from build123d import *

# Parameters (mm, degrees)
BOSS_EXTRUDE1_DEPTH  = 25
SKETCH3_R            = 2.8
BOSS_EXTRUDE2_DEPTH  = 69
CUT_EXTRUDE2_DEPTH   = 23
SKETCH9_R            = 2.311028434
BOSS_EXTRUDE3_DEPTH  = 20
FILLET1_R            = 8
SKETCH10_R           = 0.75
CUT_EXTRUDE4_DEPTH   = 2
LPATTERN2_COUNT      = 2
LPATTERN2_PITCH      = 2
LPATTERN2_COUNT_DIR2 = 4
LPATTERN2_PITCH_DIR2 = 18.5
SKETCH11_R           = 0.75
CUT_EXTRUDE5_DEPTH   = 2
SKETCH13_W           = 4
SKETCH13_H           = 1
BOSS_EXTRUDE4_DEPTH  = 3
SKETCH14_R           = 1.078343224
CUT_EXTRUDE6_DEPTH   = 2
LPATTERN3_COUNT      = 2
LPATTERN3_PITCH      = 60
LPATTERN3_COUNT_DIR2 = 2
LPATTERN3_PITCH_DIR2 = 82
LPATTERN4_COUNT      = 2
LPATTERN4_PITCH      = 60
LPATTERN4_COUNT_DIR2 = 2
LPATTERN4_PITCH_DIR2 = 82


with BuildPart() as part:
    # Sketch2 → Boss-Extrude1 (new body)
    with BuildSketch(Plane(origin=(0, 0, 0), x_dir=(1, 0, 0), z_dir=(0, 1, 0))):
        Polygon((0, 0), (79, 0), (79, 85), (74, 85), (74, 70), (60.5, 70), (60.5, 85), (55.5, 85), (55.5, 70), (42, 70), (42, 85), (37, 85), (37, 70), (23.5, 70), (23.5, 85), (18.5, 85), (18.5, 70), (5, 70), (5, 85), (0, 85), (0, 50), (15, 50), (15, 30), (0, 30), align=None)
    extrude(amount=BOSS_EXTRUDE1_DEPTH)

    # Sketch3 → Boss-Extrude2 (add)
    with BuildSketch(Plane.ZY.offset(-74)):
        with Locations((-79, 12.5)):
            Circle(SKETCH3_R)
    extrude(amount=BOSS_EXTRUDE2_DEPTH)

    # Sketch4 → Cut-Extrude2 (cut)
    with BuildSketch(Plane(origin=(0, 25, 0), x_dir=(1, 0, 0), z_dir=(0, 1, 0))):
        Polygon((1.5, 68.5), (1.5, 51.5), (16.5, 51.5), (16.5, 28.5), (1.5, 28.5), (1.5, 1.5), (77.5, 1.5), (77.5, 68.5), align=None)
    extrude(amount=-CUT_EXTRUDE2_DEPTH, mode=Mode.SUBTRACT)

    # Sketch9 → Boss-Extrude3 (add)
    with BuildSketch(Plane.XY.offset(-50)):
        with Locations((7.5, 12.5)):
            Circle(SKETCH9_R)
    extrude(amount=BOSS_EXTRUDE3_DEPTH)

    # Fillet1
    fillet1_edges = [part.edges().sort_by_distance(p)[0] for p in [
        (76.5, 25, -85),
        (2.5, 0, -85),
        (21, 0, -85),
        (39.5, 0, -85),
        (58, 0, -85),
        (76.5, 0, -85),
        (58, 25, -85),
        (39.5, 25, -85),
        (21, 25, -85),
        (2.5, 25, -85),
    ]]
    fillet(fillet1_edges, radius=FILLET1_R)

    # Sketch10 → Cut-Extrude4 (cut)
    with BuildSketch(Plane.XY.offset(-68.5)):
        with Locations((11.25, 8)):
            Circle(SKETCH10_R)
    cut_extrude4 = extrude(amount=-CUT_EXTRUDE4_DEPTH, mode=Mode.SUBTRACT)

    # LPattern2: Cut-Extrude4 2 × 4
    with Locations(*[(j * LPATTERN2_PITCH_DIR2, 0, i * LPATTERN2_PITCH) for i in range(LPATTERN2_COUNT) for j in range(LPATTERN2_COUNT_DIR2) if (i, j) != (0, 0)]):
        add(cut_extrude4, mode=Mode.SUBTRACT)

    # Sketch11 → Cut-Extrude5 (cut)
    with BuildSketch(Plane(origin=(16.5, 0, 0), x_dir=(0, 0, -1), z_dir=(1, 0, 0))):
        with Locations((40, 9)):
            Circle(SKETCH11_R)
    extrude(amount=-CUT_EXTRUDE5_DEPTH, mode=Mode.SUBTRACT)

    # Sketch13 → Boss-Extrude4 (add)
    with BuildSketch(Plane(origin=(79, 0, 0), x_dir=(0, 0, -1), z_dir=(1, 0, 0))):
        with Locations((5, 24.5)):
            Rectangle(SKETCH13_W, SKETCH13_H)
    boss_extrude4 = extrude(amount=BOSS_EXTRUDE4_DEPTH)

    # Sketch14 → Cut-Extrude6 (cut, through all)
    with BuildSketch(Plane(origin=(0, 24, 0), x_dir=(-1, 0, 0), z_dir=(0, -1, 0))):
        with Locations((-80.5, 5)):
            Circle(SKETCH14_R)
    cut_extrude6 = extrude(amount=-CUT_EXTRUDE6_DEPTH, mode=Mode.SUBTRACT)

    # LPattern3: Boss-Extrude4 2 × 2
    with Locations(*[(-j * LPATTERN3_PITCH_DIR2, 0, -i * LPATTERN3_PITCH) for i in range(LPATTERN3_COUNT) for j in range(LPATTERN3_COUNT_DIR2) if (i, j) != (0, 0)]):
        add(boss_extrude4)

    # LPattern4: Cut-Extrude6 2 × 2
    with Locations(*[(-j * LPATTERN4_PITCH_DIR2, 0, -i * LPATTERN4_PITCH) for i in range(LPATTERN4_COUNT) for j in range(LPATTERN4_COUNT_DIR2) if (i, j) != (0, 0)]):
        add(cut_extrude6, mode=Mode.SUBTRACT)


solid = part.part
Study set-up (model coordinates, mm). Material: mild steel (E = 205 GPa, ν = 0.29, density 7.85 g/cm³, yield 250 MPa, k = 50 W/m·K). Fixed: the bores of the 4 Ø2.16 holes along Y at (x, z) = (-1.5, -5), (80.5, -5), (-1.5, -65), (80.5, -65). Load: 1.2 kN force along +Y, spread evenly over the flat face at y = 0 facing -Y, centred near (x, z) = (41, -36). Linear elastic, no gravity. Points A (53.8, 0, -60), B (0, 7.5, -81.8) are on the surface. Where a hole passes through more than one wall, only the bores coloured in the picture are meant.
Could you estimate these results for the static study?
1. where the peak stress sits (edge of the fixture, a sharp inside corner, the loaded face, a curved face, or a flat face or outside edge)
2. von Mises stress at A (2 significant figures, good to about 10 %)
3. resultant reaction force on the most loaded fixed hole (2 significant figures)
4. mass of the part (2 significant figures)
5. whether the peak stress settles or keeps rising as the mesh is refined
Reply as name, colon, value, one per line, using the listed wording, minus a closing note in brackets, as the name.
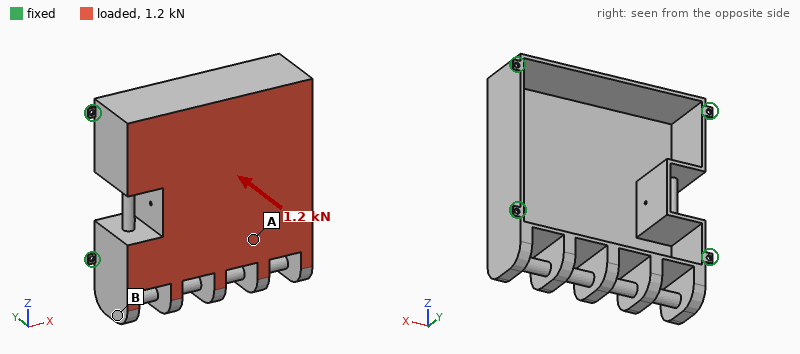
where the peak stress sits: edge of the fixture
von Mises stress at A: 22 MPa
resultant reaction force on the most loaded fixed hole: 360 N
mass of the part: 250 g
whether the peak stress settles or keeps rising as the mesh is refined: keeps rising
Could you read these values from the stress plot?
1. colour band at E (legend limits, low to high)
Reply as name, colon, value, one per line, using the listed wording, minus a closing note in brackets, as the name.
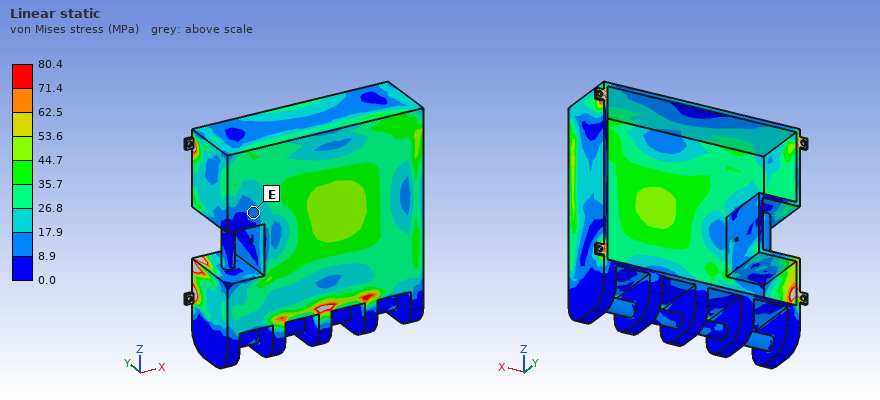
colour band at E: 8.9 to 17.9 MPa
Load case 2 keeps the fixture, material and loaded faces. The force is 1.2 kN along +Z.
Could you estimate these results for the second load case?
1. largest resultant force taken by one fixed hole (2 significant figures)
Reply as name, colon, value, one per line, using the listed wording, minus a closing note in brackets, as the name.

largest resultant force taken by one fixed hole: 590 N
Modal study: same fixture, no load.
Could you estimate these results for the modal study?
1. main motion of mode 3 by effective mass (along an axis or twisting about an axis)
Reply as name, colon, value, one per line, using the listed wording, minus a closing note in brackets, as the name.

main motion of mode 3 by effective mass: along X
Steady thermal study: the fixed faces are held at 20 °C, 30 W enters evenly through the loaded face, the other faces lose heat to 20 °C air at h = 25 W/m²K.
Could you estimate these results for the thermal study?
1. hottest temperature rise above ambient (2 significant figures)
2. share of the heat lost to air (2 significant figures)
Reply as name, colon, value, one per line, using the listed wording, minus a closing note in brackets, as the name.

hottest temperature rise above ambient: 57 K
share of the heat lost to air: 75 %
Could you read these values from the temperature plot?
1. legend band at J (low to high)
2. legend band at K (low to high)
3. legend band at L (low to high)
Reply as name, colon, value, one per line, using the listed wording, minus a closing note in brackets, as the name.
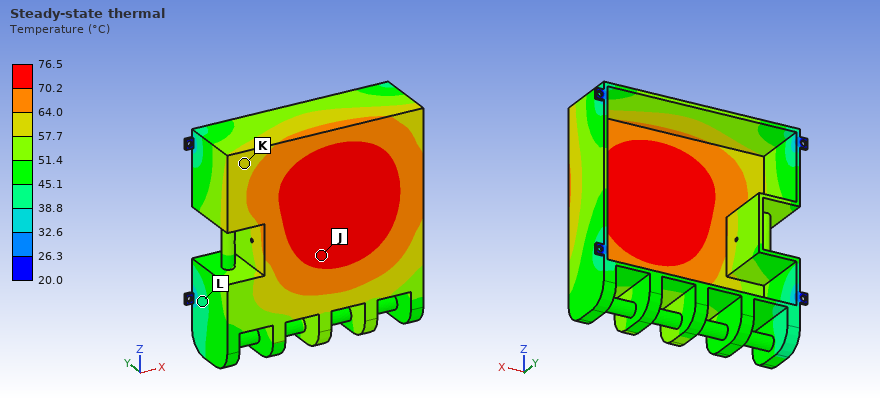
legend band at J: 70.2 to 76.5 °C
legend band at K: 57.7 to 64.0 °C
legend band at L: 38.8 to 45.1 °C
